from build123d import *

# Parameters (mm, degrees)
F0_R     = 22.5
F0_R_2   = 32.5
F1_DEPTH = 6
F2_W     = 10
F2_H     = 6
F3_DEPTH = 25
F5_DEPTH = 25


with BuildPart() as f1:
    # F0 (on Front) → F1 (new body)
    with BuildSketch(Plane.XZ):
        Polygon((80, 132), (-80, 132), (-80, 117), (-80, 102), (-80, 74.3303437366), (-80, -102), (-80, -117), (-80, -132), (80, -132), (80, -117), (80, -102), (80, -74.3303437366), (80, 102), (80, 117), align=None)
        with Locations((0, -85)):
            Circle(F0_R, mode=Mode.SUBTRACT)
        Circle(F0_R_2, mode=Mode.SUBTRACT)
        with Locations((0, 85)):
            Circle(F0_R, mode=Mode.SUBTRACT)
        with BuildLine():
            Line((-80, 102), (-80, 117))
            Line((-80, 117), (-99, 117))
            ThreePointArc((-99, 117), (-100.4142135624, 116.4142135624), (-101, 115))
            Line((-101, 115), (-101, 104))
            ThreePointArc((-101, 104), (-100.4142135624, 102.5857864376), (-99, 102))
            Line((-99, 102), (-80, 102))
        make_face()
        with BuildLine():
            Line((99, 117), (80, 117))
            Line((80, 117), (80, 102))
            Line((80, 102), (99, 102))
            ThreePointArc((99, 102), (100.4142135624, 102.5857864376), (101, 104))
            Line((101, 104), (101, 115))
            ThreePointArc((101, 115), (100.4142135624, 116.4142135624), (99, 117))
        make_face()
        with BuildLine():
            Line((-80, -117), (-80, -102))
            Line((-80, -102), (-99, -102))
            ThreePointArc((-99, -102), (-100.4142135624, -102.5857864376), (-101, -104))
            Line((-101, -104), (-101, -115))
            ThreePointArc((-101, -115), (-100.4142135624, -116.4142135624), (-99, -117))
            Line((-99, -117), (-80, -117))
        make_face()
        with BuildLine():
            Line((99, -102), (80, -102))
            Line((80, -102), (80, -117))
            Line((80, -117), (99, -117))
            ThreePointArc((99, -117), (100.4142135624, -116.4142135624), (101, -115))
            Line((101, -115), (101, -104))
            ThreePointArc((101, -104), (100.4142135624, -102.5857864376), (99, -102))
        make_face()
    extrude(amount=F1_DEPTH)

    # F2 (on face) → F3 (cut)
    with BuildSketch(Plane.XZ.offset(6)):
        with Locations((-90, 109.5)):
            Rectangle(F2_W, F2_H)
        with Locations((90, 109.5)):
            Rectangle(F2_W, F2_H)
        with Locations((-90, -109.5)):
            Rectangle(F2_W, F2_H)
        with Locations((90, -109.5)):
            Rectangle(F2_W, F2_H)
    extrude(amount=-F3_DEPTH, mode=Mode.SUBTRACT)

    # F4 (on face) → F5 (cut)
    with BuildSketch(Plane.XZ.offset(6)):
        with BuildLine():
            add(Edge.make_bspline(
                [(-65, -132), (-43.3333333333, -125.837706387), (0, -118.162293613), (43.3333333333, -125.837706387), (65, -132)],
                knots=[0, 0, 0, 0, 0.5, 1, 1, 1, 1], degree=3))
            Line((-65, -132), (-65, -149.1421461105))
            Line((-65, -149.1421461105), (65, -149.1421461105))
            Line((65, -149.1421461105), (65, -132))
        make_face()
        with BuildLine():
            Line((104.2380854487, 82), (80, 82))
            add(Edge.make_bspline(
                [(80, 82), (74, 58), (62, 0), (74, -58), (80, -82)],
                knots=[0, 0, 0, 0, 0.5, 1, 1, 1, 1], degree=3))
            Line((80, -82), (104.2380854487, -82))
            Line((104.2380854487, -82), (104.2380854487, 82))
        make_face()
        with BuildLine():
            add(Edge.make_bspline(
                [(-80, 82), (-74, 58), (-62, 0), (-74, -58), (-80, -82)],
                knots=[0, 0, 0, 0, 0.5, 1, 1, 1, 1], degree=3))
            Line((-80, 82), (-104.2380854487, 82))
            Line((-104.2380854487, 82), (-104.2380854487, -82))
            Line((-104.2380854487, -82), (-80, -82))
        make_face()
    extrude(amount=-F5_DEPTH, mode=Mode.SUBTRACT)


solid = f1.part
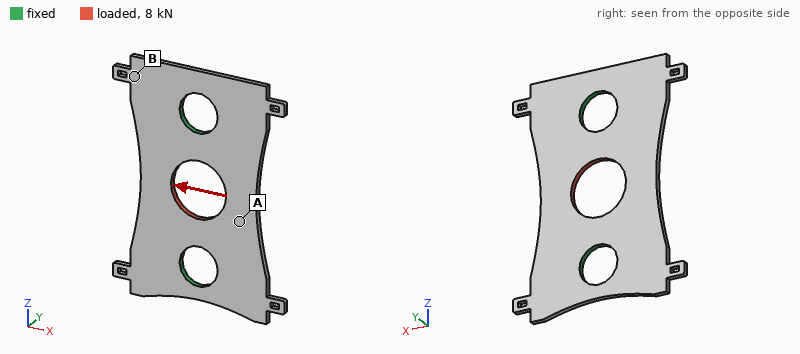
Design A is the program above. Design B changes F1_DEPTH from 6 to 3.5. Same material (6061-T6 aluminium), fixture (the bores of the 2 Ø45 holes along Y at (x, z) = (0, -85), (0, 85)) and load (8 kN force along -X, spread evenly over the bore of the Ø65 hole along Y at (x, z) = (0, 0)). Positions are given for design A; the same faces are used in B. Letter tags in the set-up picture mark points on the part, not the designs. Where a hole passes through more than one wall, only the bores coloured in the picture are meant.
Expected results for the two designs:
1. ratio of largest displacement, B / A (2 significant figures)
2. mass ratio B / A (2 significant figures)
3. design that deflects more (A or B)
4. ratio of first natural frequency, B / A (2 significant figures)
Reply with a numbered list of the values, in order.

1. 1.7
2. 0.58
3. B
4. 0.59
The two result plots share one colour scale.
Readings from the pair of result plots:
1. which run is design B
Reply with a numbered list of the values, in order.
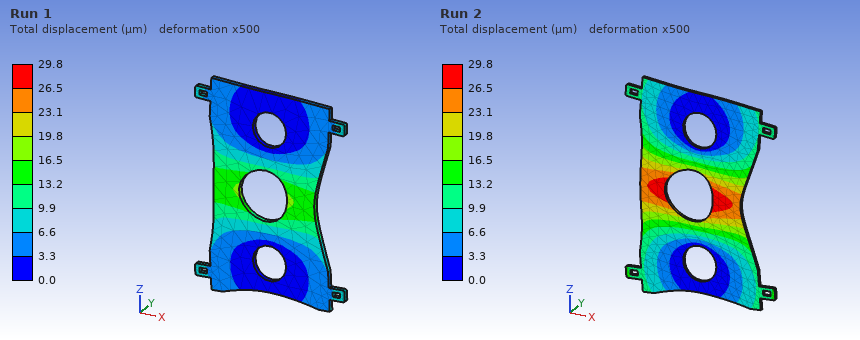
1. Run 2
